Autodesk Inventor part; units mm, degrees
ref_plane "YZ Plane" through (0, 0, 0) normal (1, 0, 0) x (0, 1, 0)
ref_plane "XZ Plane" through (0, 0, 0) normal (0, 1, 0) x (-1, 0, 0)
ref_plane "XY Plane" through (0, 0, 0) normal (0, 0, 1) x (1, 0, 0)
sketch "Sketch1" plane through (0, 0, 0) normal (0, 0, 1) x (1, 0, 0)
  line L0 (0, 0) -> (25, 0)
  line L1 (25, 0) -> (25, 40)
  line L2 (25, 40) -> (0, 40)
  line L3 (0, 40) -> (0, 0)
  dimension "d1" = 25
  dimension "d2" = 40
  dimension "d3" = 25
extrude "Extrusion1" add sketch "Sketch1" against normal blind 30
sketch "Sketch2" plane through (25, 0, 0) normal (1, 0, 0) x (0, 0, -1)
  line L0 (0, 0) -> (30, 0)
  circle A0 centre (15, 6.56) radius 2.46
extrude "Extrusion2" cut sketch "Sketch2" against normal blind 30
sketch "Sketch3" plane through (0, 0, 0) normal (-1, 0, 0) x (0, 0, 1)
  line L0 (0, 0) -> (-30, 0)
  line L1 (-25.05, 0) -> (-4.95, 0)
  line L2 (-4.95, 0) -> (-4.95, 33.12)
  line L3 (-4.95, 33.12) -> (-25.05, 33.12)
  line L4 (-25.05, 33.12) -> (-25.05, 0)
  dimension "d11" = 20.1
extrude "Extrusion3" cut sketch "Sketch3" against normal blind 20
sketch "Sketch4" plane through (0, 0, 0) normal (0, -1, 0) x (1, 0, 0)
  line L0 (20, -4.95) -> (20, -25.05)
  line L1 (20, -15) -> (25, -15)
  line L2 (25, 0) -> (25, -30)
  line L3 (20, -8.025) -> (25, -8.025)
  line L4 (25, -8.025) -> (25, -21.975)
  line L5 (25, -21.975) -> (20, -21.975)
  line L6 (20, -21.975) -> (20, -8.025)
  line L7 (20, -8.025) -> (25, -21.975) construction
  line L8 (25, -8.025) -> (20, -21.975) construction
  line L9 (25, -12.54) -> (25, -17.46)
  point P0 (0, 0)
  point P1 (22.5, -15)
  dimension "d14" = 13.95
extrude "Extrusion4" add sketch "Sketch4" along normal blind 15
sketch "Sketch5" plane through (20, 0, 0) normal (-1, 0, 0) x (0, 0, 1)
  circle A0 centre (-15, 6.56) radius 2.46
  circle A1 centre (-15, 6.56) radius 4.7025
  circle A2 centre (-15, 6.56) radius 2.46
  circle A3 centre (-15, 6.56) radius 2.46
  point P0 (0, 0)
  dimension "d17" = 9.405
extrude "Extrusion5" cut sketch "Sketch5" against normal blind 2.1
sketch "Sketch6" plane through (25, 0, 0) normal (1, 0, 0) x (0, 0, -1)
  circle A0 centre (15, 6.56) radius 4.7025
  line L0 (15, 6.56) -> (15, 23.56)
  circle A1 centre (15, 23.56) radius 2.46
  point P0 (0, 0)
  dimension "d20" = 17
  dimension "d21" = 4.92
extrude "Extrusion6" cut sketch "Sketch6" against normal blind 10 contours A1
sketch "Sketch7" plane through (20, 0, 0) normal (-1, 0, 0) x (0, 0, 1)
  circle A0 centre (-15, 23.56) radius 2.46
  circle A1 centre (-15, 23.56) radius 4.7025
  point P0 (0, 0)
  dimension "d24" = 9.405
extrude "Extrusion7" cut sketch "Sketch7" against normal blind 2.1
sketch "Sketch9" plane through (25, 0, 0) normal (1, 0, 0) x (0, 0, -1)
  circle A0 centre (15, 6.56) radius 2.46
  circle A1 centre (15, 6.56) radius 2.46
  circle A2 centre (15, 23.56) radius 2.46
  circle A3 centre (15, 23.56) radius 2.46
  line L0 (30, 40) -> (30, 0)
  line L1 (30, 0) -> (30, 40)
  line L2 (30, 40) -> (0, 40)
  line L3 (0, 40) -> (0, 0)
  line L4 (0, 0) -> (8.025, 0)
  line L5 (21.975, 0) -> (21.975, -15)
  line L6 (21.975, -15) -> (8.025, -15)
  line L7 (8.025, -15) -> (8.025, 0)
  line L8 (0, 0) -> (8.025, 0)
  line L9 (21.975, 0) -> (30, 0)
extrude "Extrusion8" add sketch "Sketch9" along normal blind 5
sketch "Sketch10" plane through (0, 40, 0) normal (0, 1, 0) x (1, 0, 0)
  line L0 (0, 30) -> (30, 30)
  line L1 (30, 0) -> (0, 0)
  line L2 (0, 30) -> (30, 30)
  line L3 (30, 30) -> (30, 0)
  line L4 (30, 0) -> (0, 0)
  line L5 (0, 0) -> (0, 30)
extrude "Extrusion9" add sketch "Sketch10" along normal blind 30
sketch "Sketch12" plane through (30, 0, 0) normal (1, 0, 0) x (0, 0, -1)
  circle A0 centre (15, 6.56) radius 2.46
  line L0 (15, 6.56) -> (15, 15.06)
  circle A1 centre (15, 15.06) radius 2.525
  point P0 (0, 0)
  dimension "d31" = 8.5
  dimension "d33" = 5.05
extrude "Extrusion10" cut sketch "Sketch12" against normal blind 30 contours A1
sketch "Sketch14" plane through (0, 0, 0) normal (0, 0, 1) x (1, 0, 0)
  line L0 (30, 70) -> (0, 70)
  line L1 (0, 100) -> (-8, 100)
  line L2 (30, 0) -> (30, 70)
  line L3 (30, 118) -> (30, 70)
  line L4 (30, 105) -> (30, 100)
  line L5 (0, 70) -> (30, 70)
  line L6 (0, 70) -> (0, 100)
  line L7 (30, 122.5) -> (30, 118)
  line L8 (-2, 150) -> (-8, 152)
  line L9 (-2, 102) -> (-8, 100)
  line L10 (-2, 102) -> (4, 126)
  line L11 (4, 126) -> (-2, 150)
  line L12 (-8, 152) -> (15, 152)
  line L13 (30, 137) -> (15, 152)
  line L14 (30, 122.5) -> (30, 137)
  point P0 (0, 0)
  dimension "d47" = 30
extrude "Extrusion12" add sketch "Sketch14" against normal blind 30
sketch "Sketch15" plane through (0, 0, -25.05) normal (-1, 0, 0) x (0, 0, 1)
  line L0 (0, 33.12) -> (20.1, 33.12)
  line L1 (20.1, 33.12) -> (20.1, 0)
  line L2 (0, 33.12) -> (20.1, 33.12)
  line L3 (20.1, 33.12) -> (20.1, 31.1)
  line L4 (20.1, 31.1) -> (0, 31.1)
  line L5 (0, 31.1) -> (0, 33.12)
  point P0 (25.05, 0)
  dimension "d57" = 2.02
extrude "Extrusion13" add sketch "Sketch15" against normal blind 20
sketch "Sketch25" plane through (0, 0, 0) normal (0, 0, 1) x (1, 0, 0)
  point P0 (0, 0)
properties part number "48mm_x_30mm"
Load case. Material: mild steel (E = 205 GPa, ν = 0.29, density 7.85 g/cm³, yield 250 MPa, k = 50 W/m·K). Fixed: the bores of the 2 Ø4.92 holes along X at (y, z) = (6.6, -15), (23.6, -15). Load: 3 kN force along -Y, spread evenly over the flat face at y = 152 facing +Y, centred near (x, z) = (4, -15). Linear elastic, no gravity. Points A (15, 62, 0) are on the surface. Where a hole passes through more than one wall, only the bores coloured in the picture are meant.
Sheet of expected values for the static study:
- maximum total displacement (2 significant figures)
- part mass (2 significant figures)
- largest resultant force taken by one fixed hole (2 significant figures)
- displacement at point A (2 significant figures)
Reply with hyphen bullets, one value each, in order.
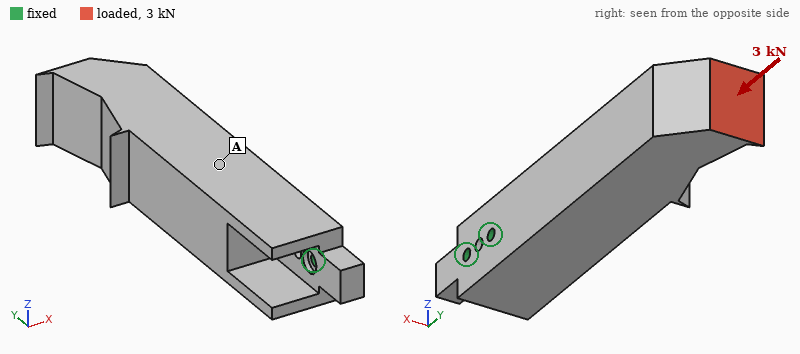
- 97 µm
- 950 g
- 3.1 kN
- 20 µm
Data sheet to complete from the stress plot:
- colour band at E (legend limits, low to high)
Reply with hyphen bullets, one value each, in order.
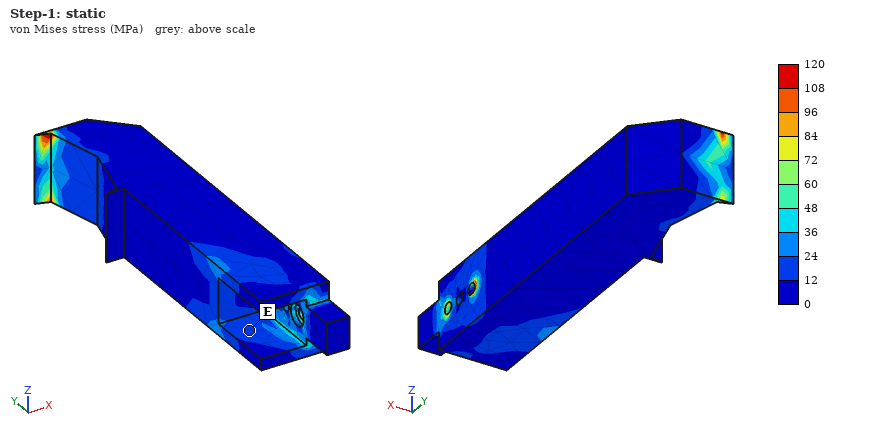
- 12 to 24 MPa
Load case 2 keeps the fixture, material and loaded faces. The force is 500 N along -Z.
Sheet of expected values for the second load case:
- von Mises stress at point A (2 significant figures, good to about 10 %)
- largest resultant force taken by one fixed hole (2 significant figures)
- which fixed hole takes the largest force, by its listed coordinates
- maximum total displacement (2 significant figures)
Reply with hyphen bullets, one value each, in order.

- 10 MPa
- 3.3 kN
- (23.6, -15)
- 68 µm
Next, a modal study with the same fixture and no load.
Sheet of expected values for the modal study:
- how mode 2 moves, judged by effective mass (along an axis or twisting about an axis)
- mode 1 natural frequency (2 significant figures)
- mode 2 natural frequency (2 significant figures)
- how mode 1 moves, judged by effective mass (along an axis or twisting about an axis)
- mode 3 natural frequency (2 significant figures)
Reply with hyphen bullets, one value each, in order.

- along Z
- 770 Hz
- 900 Hz
- along X
- 2900 Hz
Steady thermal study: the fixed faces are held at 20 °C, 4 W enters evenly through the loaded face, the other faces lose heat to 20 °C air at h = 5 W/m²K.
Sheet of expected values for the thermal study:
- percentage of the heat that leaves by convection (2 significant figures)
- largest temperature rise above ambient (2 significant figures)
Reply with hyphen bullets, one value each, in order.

- 15 %
- 17 K
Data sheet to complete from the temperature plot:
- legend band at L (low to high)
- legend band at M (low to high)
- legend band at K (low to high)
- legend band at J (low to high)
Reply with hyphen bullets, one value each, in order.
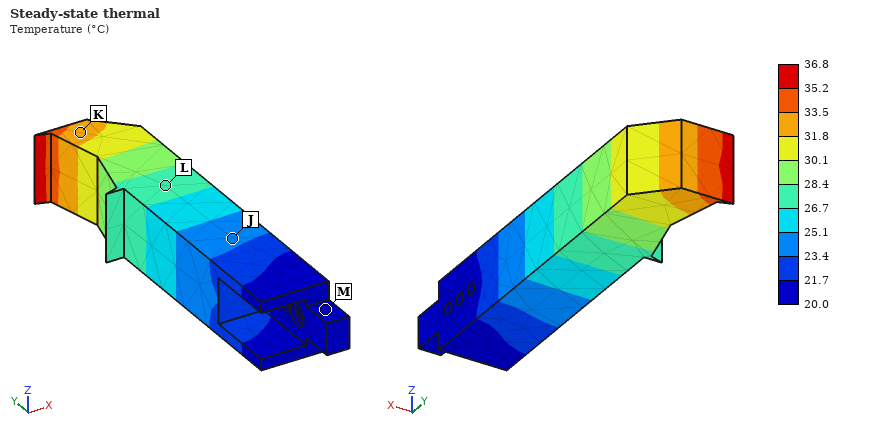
- 26.7 to 28.4 °C
- 20.0 to 21.7 °C
- 31.8 to 33.5 °C
- 23.4 to 25.1 °C
